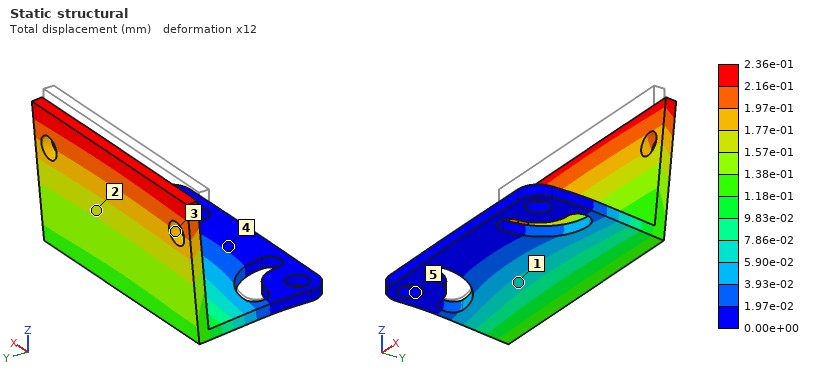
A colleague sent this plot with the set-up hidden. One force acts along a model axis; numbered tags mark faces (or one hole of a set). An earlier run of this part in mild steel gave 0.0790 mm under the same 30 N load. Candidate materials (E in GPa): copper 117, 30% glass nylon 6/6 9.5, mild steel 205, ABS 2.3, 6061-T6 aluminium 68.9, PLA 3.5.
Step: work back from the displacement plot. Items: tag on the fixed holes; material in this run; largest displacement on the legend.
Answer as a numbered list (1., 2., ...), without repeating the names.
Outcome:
1. 5
2. 6061-T6 aluminium
3. 2.36e-01 mm
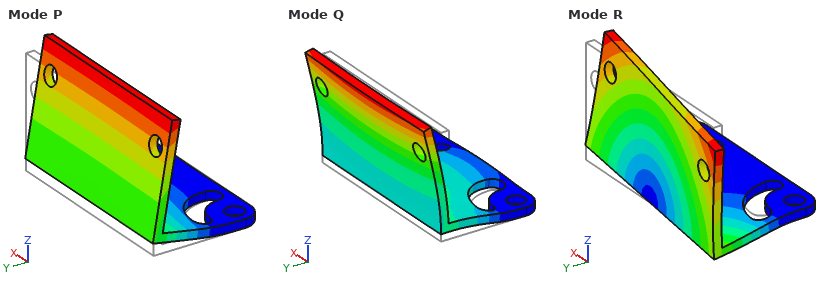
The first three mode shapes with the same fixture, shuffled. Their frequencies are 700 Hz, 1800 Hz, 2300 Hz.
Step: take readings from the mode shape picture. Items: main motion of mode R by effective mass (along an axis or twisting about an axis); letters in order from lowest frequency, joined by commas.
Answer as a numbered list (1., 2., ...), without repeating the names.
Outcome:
1. along X
2. P, R, Q
